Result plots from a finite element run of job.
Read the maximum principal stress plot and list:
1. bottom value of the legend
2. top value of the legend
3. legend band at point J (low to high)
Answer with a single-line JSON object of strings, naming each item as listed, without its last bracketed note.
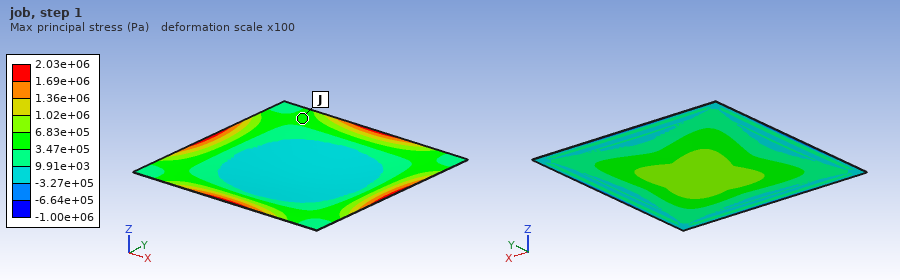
{"bottom value of the legend": "-1.00e+06 Pa", "top value of the legend": "2.03e+06 Pa", "legend band at point J": "3.47e+05 to 6.83e+05 Pa"}
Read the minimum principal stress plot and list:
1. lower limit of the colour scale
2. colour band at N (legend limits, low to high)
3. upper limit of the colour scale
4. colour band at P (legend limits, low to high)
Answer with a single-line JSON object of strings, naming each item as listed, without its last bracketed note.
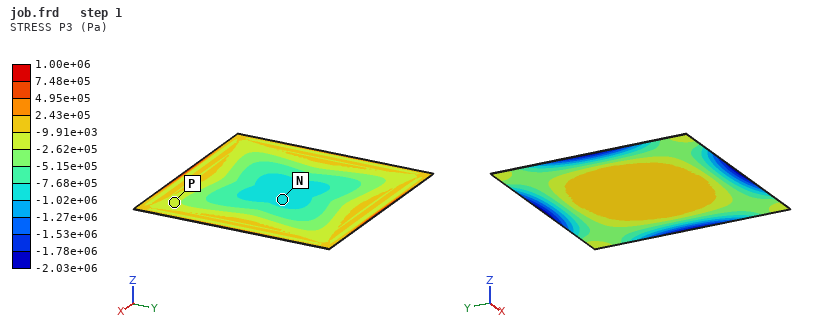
{"lower limit of the colour scale": "-2.03e+06 Pa", "colour band at N": "-1.02e+06 to -7.68e+05 Pa", "upper limit of the colour scale": "1.00e+06 Pa", "colour band at P": "-2.62e+05 to -9.91e+03 Pa"}
